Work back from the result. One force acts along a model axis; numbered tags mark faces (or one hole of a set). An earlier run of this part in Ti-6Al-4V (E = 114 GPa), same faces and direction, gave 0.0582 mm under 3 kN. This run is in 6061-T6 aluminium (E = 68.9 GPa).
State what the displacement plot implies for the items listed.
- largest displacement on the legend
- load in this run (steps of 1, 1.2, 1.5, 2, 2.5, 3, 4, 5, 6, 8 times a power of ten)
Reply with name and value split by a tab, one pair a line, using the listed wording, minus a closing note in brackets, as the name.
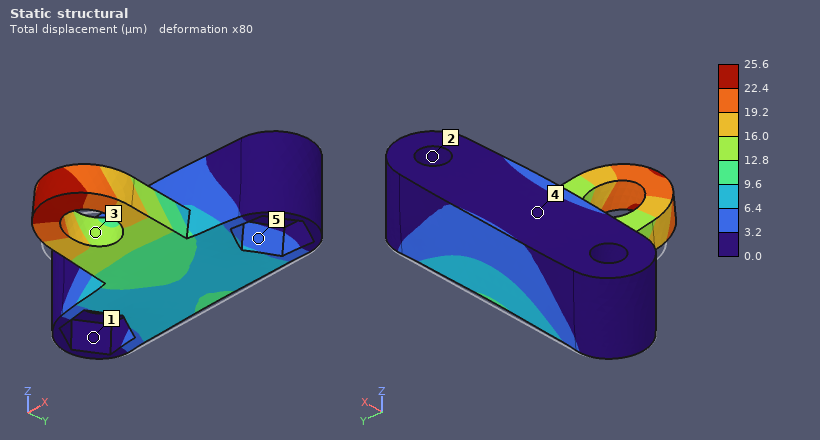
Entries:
largest displacement on the legend	25.6 µm
load in this run	800 N
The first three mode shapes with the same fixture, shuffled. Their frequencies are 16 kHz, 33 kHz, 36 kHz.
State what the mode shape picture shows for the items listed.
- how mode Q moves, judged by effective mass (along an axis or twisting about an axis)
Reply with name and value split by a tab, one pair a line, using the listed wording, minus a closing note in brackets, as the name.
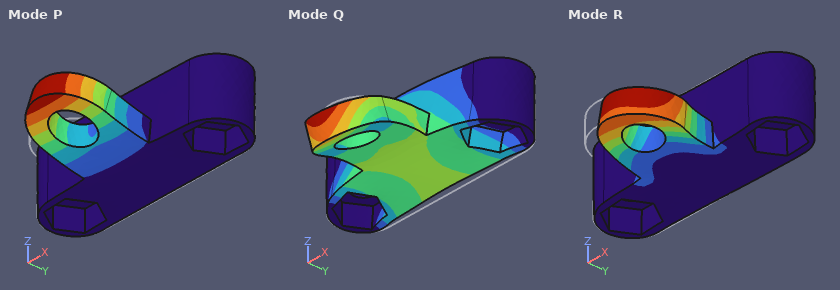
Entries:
how mode Q moves, judged by effective mass	along Y
